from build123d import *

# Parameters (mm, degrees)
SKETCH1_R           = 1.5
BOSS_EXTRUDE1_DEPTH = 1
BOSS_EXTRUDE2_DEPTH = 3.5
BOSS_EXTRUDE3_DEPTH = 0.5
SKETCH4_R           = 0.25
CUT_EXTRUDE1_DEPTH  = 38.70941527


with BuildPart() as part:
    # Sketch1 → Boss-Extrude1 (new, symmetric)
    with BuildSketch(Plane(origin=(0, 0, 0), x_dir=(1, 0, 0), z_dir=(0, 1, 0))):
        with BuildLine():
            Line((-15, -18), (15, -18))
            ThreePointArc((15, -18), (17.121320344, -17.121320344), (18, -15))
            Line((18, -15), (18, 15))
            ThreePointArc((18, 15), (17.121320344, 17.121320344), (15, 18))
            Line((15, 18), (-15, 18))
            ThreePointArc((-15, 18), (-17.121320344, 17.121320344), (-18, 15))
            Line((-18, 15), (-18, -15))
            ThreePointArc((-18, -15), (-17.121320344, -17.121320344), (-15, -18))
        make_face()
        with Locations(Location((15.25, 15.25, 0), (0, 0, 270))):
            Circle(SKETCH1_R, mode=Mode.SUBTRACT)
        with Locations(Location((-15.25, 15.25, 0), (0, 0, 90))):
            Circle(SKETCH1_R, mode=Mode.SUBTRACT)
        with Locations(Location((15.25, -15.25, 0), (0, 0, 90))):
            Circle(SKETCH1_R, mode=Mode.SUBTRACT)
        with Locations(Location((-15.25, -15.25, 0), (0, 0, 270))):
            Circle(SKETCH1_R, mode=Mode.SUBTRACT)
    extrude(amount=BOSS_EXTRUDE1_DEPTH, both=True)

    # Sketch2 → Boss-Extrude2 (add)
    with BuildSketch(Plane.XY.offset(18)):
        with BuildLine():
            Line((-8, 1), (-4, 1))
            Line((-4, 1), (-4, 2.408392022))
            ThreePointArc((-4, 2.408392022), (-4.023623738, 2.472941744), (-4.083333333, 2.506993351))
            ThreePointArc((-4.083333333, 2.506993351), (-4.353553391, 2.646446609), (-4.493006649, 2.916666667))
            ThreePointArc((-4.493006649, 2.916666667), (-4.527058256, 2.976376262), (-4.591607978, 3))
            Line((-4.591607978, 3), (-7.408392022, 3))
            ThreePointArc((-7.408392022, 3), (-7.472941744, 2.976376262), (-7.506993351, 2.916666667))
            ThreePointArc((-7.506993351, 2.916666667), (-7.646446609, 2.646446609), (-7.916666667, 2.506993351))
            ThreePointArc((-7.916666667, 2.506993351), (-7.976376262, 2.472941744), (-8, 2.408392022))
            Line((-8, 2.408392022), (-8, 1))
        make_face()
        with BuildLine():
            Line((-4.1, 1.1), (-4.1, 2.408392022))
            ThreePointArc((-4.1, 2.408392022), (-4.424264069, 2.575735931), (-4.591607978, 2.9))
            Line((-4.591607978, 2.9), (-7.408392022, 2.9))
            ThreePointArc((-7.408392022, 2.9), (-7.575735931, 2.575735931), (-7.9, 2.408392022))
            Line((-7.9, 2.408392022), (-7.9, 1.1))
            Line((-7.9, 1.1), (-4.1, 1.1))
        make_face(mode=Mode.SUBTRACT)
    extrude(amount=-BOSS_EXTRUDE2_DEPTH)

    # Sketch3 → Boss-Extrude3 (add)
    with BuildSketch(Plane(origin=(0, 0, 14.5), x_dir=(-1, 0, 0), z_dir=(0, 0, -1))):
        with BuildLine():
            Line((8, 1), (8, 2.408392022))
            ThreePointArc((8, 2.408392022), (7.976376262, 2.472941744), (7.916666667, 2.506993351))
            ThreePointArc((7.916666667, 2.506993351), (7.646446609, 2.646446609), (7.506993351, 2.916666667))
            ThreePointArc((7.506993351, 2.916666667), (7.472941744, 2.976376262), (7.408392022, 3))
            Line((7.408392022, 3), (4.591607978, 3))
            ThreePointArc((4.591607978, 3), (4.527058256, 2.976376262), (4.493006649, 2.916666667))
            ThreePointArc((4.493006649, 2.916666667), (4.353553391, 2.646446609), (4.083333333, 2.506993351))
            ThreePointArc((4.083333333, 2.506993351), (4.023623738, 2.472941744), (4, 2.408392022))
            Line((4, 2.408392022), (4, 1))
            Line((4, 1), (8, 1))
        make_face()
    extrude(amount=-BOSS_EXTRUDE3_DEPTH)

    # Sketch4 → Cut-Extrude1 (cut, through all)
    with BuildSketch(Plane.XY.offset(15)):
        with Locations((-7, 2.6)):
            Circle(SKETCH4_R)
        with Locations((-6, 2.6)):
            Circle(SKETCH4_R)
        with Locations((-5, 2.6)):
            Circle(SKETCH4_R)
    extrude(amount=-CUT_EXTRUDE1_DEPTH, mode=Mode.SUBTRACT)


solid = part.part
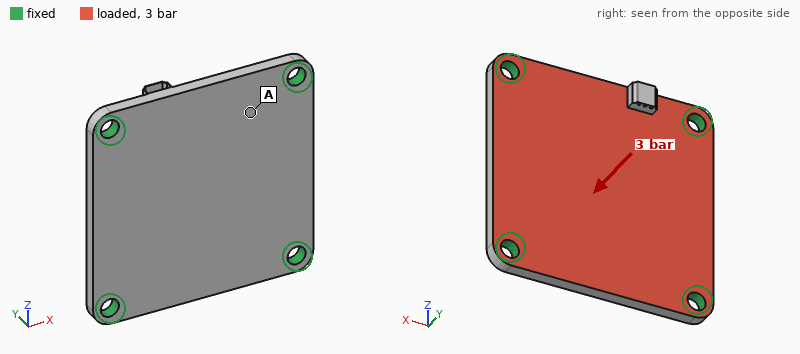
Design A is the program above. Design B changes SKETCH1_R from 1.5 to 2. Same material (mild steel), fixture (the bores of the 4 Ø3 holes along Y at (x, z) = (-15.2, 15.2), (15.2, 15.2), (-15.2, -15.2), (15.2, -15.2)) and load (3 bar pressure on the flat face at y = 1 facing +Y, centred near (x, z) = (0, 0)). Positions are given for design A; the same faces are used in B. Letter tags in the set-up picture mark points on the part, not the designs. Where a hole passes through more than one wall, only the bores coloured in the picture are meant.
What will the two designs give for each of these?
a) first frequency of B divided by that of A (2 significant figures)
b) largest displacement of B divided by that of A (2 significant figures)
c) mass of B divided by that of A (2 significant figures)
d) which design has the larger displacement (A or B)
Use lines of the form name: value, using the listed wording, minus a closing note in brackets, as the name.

first frequency of B divided by that of A: 1.1
largest displacement of B divided by that of A: 0.86
mass of B divided by that of A: 0.98
which design has the larger displacement: A
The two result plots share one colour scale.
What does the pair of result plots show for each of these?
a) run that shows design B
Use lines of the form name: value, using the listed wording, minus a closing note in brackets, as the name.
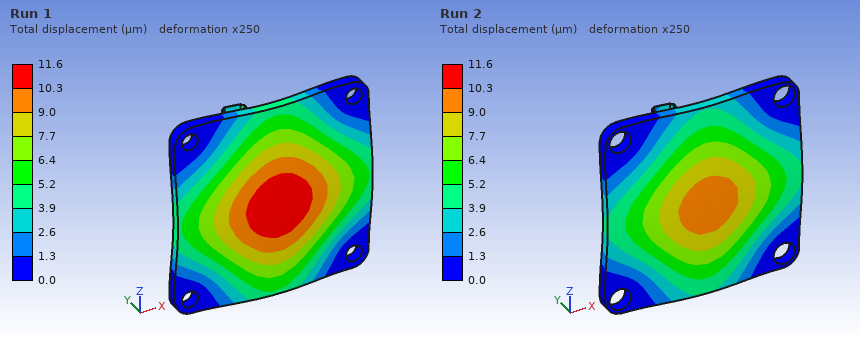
run that shows design B: Run 2
